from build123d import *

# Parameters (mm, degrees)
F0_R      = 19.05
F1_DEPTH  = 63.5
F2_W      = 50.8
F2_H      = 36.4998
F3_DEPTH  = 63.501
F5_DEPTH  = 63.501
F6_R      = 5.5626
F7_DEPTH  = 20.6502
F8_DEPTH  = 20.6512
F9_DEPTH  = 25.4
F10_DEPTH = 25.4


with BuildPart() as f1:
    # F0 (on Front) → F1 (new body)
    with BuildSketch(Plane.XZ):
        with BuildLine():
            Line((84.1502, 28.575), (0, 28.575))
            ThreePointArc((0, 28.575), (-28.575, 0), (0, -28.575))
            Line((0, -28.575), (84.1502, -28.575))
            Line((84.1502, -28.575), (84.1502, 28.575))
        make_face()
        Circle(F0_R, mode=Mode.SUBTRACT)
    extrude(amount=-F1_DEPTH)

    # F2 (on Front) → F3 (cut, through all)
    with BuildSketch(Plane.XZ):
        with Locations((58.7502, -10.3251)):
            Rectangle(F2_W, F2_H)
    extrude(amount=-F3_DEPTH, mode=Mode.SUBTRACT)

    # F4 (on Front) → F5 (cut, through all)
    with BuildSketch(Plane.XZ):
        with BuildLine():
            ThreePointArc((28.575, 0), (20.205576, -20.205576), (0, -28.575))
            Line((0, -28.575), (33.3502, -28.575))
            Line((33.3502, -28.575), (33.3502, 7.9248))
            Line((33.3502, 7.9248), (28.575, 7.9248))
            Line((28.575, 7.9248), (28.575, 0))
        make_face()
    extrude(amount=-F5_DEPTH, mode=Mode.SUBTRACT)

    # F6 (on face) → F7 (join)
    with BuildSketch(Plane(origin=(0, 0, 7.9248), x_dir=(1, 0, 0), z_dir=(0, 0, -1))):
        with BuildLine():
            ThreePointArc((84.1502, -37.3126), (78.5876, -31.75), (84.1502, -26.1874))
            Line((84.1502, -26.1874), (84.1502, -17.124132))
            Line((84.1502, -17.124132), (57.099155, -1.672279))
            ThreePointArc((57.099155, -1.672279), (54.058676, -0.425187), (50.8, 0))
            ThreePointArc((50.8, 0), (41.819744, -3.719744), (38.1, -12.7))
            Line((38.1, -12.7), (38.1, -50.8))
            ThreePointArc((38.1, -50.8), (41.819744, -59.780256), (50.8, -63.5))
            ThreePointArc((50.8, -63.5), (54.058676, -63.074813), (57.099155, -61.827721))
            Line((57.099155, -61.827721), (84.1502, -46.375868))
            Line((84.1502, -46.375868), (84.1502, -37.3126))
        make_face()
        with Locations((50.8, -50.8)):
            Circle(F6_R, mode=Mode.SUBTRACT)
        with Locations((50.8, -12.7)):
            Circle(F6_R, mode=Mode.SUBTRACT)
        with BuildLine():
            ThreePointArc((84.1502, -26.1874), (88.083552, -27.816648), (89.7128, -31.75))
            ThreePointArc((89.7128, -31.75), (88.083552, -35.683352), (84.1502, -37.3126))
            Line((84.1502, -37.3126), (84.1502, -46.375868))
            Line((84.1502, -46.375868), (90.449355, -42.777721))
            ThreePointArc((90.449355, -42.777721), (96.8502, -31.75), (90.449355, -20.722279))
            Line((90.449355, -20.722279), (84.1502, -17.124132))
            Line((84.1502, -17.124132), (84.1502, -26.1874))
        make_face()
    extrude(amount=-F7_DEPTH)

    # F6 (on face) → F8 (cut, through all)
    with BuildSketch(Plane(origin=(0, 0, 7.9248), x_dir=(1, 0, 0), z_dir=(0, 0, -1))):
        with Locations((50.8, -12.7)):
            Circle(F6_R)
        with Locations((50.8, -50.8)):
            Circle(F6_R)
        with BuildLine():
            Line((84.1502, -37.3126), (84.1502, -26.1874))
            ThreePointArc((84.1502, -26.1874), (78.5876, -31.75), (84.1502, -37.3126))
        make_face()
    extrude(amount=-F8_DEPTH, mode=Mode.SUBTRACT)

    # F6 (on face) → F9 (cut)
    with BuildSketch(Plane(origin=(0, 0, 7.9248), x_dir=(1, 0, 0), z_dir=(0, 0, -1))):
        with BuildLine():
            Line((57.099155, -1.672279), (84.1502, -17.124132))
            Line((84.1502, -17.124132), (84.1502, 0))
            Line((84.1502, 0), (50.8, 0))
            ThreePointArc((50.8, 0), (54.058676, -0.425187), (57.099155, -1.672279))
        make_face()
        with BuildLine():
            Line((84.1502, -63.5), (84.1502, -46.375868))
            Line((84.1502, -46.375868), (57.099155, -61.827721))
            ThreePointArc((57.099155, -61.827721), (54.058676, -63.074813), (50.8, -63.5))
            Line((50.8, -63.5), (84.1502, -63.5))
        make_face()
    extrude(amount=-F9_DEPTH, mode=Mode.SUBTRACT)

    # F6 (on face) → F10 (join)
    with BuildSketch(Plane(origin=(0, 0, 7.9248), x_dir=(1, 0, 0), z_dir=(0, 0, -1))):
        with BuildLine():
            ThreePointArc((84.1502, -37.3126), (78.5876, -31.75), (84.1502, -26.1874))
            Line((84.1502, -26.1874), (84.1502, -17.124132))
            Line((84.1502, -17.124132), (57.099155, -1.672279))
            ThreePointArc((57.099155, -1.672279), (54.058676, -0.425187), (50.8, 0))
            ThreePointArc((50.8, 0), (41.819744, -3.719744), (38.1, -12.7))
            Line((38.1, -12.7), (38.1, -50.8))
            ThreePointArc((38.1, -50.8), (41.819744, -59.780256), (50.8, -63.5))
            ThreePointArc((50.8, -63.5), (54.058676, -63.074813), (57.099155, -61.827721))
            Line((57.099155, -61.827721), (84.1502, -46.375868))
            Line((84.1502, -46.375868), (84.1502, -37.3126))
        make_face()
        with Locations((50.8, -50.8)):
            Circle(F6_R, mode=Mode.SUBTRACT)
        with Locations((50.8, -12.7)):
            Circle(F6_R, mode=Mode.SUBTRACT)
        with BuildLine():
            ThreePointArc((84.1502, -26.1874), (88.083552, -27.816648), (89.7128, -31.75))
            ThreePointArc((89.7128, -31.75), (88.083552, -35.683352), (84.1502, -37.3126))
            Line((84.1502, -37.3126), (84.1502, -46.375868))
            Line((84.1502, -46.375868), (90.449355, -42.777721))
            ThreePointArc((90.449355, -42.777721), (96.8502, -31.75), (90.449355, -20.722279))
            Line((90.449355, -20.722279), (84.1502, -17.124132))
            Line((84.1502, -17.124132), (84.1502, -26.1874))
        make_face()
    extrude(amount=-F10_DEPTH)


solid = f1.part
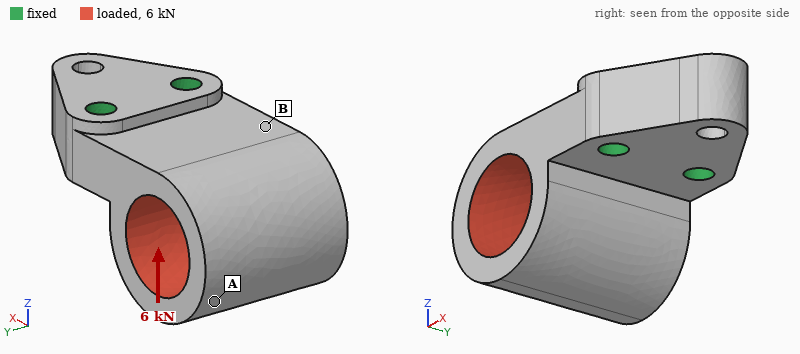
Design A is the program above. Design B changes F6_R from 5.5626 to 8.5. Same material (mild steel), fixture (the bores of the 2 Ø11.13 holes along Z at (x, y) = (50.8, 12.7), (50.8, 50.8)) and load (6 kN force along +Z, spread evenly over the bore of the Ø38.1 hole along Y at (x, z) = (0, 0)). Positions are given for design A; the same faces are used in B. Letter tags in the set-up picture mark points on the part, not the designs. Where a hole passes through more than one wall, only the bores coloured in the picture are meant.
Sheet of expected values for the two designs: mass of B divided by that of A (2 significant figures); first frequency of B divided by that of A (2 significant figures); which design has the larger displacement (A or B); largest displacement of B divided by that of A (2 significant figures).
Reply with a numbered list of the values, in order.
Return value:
1. 0.96
2. 1.1
3. A
4. 0.89
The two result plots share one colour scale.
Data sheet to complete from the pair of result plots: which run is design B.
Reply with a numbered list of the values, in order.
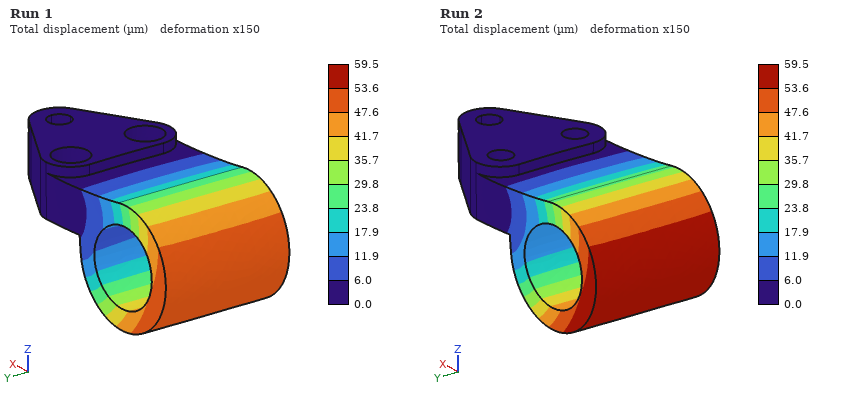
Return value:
1. Run 1
